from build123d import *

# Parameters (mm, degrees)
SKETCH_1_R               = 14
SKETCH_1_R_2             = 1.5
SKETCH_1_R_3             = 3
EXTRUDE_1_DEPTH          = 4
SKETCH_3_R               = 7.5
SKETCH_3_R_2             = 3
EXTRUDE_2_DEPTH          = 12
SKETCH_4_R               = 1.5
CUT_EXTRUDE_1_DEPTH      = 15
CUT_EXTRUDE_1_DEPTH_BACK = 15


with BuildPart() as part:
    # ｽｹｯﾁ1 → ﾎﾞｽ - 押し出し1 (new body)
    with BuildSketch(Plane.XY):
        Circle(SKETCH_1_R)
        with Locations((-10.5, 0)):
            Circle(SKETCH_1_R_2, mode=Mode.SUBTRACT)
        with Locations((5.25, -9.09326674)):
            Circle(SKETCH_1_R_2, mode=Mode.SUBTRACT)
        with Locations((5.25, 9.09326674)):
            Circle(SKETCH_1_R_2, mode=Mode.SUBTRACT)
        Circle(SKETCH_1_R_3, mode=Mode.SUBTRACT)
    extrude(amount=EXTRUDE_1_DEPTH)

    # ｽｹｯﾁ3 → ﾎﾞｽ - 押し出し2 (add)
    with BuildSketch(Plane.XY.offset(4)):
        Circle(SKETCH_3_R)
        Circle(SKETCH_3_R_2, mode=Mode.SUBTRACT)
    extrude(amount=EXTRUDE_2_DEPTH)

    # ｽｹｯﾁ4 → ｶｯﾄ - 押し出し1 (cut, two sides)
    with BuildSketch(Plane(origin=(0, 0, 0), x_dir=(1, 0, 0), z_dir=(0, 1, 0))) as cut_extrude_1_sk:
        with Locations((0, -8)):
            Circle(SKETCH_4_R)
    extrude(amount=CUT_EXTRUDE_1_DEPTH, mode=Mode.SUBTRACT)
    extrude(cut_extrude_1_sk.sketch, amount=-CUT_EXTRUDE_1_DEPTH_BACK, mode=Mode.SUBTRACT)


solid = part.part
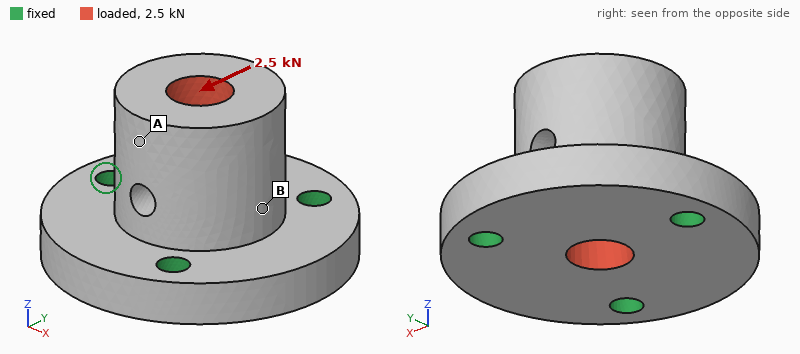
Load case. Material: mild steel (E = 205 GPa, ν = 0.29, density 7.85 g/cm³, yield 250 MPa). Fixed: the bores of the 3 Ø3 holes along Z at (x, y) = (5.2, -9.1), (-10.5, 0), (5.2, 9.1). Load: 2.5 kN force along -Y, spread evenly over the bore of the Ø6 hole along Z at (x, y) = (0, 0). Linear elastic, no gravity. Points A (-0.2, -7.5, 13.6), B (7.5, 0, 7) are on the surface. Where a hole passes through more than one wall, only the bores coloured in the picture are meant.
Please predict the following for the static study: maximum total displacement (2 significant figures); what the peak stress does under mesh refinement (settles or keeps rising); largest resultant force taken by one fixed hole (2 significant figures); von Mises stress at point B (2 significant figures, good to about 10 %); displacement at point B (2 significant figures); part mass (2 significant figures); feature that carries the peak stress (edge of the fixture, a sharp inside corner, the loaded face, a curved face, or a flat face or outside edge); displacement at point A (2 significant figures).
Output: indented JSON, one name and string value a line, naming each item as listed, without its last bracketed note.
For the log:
{
  "maximum total displacement": "7.3 µm",
  "what the peak stress does under mesh refinement": "keeps rising",
  "largest resultant force taken by one fixed hole": "1.2 kN",
  "von Mises stress at point B": "21 MPa",
  "displacement at point B": "2.2 µm",
  "part mass": "31 g",
  "feature that carries the peak stress": "edge of the fixture",
  "displacement at point A": "6.3 µm"
}
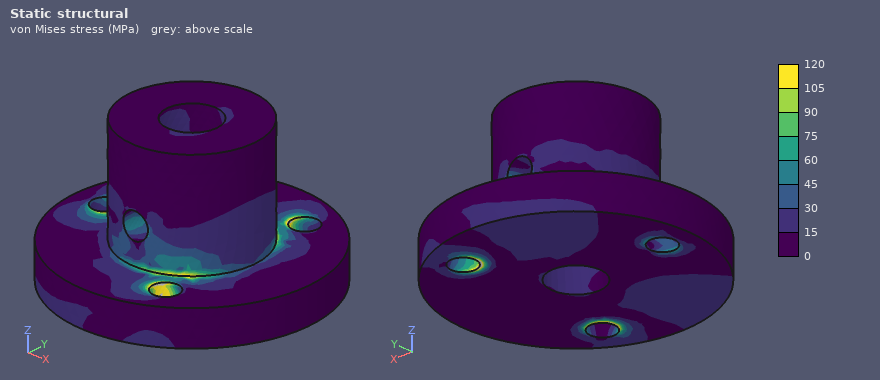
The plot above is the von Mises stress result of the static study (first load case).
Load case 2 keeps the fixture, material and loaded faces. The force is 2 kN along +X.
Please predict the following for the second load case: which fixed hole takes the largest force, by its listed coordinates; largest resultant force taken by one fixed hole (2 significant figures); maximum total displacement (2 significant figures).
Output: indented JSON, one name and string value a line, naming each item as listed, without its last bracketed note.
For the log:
{
  "which fixed hole takes the largest force, by its listed coordinates": "(-10.5, 0)",
  "largest resultant force taken by one fixed hole": "1.1 kN",
  "maximum total displacement": "5.9 µm"
}
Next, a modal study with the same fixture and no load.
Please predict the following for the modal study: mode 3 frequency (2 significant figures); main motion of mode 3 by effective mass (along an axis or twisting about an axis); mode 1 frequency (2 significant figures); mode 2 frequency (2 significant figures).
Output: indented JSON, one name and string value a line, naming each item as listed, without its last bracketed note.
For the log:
{
  "mode 3 frequency": "35 kHz",
  "main motion of mode 3 by effective mass": "along Z",
  "mode 1 frequency": "24 kHz",
  "mode 2 frequency": "25 kHz"
}
